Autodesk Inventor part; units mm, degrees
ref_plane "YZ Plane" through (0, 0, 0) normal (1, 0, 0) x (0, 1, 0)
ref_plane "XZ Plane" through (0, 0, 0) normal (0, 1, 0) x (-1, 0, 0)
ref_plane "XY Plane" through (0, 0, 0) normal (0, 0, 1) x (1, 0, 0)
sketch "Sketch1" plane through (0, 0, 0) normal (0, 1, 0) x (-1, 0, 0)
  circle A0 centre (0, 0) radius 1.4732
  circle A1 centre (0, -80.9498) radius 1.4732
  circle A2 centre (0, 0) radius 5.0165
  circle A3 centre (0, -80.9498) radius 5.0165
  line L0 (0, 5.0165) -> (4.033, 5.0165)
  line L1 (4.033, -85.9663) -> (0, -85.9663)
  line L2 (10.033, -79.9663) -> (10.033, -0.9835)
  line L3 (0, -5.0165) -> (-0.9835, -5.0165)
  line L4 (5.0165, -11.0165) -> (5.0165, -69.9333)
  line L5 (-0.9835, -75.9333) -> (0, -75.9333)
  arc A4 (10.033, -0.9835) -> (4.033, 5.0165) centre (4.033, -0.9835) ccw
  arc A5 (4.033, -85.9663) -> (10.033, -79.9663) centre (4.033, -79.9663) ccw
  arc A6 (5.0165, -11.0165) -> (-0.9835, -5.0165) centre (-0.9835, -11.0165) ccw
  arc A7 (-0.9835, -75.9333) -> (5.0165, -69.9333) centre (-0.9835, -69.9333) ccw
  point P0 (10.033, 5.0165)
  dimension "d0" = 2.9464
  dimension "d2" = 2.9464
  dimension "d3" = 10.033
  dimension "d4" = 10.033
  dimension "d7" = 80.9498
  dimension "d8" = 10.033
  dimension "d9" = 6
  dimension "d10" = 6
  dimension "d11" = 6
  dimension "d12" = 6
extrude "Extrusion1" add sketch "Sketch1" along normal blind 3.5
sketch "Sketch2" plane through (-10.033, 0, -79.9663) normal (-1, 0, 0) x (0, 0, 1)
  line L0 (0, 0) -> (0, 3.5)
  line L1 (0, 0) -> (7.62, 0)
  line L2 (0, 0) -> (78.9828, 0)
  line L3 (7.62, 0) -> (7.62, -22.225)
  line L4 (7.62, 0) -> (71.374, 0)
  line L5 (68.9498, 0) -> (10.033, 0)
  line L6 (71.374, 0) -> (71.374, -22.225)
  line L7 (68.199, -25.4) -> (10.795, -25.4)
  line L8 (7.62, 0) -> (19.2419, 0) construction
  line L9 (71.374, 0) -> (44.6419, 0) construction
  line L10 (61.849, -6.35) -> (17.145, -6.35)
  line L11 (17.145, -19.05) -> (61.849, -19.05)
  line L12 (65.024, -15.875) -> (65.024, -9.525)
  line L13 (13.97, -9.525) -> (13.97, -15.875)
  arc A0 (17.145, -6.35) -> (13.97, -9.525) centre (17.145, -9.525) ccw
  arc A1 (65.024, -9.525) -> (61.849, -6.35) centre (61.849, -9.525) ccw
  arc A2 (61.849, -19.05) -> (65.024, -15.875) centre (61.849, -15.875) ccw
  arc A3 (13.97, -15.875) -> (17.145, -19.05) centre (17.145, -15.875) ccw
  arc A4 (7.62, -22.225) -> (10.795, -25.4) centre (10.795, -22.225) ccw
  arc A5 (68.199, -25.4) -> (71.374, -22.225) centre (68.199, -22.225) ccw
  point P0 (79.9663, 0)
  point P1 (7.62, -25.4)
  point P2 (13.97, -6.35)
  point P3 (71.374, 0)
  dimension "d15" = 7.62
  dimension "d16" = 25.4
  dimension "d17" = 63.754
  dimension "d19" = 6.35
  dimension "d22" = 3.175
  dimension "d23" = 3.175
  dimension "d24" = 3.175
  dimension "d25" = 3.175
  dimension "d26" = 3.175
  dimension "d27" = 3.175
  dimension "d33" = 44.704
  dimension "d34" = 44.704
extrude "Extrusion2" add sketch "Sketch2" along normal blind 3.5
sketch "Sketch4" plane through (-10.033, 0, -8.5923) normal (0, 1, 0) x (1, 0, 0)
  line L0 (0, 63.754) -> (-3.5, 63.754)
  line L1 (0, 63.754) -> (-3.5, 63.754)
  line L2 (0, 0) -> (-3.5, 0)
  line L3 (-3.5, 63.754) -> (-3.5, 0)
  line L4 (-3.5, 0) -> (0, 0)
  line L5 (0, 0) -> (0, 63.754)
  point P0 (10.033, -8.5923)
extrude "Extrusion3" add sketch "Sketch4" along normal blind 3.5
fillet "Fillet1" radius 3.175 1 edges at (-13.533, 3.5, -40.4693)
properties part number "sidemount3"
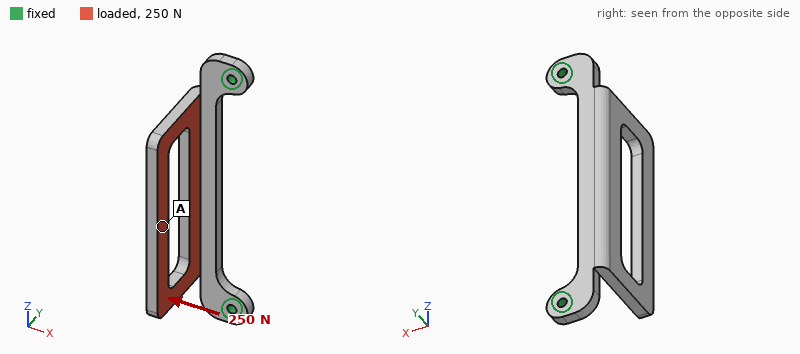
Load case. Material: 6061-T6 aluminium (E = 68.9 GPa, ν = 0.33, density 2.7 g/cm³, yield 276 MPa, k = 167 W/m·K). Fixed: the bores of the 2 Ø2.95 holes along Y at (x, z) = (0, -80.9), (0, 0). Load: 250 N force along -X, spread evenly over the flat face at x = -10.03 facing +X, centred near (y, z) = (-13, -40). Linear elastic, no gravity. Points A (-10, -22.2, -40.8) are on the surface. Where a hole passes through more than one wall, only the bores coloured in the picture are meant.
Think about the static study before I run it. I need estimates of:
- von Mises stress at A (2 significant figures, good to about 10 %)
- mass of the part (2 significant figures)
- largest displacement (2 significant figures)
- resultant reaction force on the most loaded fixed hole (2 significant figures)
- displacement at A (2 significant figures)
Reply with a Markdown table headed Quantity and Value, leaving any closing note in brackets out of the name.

| Quantity | Value |
|---|---|
| von Mises stress at A | 32 MPa |
| mass of the part | 17 g |
| largest displacement | 0.67 mm |
| resultant reaction force on the most loaded fixed hole | 210 N |
| displacement at A | 0.58 mm |
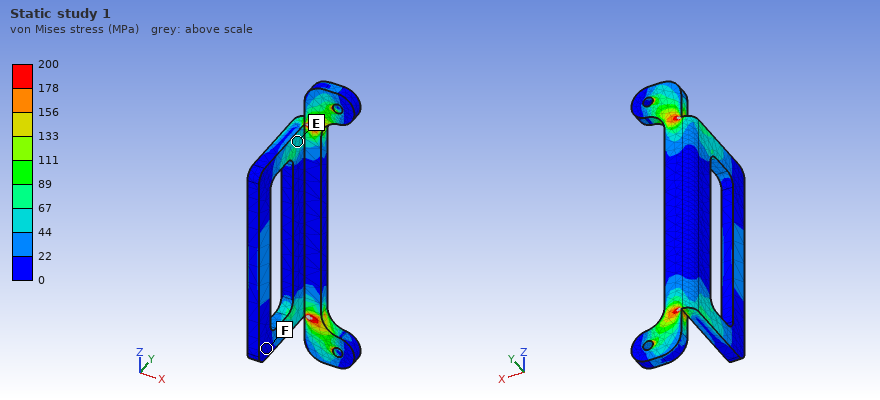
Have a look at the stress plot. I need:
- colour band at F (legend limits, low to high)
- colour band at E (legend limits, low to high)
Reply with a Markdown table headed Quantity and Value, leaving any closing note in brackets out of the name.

| Quantity | Value |
|---|---|
| colour band at F | 0 to 22 MPa |
| colour band at E | 44 to 67 MPa |
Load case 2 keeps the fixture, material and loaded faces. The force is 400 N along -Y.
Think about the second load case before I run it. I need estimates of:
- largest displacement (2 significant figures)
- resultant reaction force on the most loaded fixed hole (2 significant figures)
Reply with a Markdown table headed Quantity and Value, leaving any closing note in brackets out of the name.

| Quantity | Value |
|---|---|
| largest displacement | 0.17 mm |
| resultant reaction force on the most loaded fixed hole | 200 N |
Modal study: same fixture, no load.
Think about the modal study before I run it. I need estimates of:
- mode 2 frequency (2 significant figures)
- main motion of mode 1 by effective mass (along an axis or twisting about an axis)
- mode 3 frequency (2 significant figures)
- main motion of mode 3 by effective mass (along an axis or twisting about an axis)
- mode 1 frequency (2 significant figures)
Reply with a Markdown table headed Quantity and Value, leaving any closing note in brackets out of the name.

| Quantity | Value |
|---|---|
| mode 2 frequency | 3100 Hz |
| main motion of mode 1 by effective mass | along X |
| mode 3 frequency | 3400 Hz |
| main motion of mode 3 by effective mass | along Y |
| mode 1 frequency | 1200 Hz |
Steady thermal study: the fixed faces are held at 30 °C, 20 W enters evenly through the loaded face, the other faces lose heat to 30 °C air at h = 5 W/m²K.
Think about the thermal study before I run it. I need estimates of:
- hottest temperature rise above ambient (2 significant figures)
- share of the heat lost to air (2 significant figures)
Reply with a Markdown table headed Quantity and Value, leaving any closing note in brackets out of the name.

| Quantity | Value |
|---|---|
| hottest temperature rise above ambient | 74 K |
| share of the heat lost to air | 3.9 % |
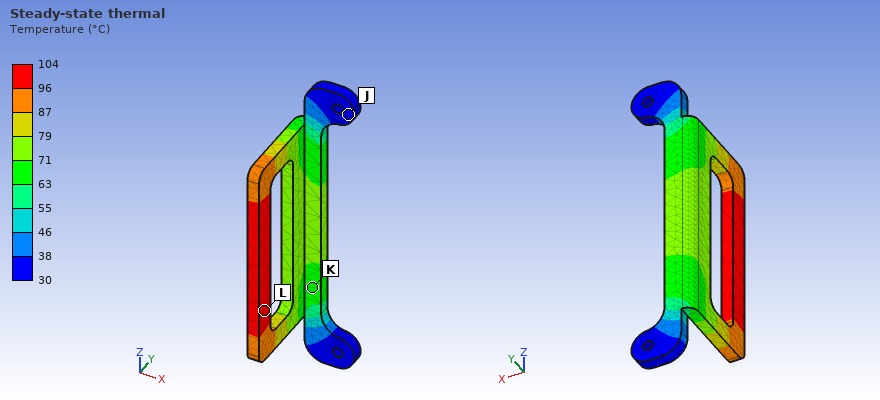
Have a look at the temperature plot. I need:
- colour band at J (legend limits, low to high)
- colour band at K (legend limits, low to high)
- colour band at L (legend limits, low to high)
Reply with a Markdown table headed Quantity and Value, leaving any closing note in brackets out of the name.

| Quantity | Value |
|---|---|
| colour band at J | 30 to 38 °C |
| colour band at K | 63 to 71 °C |
| colour band at L | 96 to 104 °C |
